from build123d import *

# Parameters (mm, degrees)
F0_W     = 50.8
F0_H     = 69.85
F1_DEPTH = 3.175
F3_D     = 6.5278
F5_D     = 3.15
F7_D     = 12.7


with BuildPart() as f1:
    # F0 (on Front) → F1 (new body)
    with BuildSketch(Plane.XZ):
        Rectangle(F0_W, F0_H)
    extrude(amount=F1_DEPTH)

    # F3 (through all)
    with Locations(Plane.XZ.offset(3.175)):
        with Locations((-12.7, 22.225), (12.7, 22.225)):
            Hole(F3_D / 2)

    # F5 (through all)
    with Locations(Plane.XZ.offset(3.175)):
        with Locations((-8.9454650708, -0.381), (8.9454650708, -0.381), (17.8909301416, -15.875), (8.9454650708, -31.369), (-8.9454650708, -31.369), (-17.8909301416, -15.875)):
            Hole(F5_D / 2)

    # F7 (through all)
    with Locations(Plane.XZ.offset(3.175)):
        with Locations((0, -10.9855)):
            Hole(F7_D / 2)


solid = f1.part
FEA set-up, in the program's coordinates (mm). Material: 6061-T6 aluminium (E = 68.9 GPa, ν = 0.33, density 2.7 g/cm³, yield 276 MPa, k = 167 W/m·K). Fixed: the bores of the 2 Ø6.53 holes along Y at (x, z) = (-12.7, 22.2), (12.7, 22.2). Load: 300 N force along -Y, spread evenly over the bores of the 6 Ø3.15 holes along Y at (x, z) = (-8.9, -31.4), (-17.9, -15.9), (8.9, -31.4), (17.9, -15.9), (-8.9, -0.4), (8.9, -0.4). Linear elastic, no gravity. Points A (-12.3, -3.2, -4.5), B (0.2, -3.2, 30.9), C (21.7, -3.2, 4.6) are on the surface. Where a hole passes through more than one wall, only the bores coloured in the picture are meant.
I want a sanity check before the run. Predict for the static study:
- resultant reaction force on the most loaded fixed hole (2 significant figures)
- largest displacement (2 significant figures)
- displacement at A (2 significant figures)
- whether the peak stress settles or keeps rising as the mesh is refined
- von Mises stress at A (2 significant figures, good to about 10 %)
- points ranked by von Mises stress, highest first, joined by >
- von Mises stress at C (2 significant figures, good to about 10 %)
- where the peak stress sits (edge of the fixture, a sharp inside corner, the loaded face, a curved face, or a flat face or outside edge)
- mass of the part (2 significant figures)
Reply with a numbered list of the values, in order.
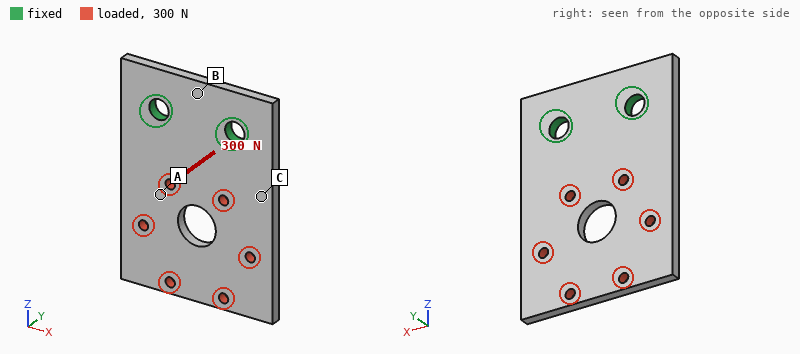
1. 150 N
2. 1.0 mm
3. 0.29 mm
4. keeps rising
5. 50 MPa
6. C > A > B
7. 76 MPa
8. edge of the fixture
9. 28 g
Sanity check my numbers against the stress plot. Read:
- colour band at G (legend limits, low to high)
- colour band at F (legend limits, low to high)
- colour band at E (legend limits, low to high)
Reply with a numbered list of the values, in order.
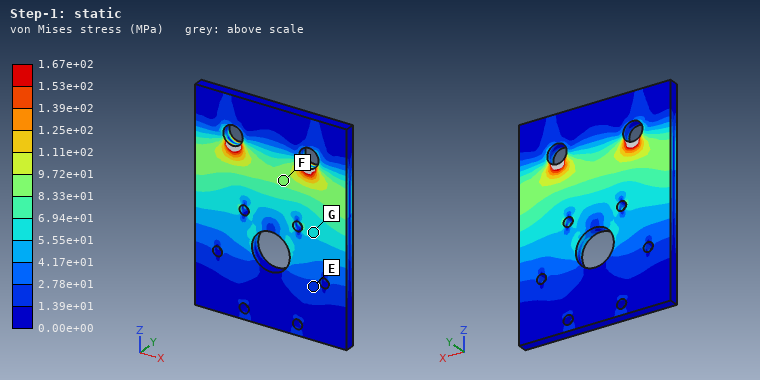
1. 5.55e+01 to 6.94e+01 MPa
2. 8.33e+01 to 9.72e+01 MPa
3. 1.39e+01 to 2.78e+01 MPa
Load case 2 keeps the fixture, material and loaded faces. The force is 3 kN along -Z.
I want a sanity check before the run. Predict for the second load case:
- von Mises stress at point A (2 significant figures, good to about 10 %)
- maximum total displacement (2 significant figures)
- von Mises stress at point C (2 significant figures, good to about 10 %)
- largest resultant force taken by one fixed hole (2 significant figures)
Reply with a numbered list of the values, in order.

1. 21 MPa
2. 16 µm
3. 16 MPa
4. 1.5 kN
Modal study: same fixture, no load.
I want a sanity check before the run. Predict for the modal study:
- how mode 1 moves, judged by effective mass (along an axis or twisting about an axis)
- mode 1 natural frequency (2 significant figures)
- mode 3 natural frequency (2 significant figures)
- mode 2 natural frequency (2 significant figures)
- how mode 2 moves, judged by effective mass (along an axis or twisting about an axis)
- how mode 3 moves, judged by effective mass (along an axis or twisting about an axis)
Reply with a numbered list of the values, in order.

1. along Y
2. 860 Hz
3. 4900 Hz
4. 2000 Hz
5. twisting about Z
6. along Y
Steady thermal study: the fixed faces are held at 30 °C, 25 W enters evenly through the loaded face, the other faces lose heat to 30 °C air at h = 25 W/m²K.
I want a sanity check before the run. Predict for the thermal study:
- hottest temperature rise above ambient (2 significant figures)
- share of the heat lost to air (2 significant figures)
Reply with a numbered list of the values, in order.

1. 37 K
2. 13 %
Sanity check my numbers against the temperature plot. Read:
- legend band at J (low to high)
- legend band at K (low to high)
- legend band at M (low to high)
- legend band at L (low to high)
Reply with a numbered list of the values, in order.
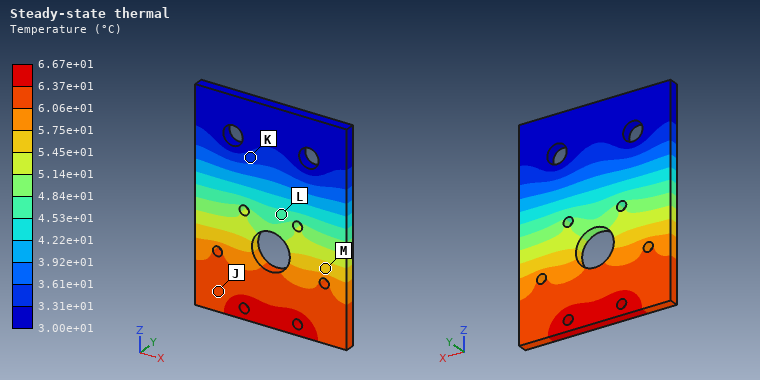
1. 6.06e+01 to 6.37e+01 °C
2. 3.31e+01 to 3.61e+01 °C
3. 5.45e+01 to 5.75e+01 °C
4. 4.53e+01 to 4.84e+01 °C
